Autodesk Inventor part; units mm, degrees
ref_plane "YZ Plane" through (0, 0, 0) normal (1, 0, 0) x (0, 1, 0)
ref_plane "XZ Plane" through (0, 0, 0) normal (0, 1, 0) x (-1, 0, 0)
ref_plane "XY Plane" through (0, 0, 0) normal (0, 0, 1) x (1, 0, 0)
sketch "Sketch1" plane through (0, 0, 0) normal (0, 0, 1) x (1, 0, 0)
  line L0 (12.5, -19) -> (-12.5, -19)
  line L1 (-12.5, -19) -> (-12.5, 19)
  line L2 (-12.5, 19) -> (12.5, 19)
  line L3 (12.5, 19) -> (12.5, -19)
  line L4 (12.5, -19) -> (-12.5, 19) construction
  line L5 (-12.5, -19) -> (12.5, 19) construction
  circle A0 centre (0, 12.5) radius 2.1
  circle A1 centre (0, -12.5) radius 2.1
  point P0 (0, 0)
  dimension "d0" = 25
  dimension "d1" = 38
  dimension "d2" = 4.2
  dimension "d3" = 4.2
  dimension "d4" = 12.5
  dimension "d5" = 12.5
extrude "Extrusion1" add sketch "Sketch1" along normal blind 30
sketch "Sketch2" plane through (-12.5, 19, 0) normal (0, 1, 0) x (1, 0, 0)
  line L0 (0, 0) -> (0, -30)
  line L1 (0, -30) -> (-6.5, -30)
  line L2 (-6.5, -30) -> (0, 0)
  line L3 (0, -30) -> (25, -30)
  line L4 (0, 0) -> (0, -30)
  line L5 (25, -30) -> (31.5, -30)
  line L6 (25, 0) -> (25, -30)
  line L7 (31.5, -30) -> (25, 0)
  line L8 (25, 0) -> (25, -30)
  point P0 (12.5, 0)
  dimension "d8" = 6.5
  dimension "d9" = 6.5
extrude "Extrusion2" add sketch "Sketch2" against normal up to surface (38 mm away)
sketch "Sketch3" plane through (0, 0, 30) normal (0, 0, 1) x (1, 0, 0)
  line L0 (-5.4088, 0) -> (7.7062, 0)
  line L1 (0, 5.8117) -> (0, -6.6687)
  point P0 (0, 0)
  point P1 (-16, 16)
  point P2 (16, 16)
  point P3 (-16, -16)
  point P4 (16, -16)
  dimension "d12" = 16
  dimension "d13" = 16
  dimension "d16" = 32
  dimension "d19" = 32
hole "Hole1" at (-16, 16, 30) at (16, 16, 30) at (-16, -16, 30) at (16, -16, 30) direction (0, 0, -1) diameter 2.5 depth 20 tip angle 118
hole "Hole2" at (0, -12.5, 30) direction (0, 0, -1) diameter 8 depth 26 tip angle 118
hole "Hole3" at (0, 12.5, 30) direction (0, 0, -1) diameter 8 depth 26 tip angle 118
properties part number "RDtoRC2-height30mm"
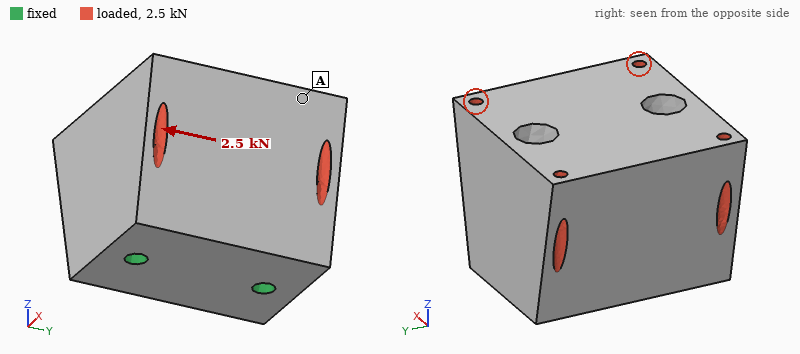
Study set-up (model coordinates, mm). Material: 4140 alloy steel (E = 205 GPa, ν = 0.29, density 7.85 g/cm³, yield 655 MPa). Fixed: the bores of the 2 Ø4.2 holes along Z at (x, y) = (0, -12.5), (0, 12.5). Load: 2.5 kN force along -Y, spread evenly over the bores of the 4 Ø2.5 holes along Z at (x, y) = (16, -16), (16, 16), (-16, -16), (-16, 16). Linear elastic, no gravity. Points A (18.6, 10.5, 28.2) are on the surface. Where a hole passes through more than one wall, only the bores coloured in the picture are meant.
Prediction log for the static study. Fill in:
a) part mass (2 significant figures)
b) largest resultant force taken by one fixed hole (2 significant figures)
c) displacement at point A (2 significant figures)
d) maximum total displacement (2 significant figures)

260 g
2.4 kN
6.1 µm
7.1 µm
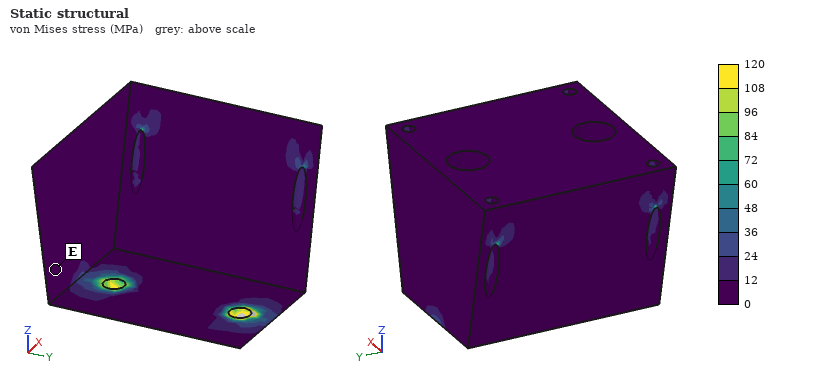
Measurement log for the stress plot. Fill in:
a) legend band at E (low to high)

0 to 12 MPa
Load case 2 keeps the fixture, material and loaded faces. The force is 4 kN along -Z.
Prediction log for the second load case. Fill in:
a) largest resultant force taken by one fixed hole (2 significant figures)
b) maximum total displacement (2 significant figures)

2.0 kN
3.8 µm
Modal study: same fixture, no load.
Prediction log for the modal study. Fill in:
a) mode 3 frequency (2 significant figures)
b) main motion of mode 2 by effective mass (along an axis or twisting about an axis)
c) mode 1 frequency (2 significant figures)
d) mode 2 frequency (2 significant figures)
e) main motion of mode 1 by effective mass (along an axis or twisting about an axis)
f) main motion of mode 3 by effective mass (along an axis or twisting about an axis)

13 kHz
along Y
2200 Hz
8200 Hz
along X
twisting about Z
